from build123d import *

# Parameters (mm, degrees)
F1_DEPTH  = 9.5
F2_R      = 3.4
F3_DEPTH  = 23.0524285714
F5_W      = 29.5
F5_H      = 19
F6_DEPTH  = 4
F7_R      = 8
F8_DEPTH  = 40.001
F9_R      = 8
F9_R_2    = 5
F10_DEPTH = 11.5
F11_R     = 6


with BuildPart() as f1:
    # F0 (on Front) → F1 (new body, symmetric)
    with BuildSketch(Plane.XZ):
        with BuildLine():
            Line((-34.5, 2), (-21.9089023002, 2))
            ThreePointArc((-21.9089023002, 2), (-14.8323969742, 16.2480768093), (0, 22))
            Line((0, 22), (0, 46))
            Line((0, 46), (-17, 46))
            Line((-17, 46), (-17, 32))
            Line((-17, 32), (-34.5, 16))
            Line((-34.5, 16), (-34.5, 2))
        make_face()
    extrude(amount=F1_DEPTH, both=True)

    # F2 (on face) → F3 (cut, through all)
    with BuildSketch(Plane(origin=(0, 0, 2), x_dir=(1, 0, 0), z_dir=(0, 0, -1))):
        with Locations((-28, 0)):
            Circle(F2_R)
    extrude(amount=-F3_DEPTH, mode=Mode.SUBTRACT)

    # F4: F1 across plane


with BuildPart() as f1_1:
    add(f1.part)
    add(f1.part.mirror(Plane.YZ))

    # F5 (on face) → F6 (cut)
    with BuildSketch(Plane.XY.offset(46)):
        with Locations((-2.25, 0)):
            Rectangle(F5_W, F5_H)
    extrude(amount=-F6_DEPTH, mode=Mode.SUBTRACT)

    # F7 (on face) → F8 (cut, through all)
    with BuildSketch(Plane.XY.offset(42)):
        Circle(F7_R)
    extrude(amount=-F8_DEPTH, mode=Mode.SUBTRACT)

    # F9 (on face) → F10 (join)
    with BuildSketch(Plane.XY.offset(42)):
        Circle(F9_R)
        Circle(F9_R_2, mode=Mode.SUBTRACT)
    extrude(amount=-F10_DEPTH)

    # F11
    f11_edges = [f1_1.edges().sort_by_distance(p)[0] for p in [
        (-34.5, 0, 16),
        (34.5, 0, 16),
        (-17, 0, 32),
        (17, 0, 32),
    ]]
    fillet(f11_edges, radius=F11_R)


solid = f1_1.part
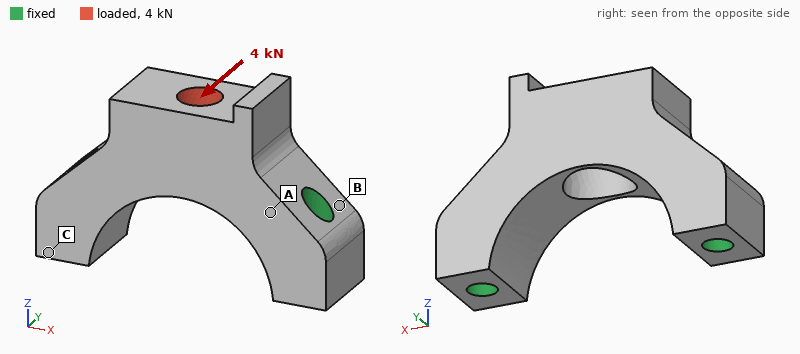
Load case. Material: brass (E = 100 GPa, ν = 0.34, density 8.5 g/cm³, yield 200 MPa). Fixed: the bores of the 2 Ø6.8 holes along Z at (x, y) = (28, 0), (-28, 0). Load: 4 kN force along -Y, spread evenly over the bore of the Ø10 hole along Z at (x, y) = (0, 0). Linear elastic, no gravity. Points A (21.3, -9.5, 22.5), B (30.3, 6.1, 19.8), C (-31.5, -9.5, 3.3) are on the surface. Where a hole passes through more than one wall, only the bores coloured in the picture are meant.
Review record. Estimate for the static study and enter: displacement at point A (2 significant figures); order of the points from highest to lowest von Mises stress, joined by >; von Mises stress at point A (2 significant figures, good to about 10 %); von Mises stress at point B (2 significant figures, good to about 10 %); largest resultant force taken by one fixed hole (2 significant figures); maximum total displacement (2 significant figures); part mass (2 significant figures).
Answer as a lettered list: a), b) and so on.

a) 7.8 µm
b) A > B > C
c) 48 MPa
d) 22 MPa
e) 2.0 kN
f) 37 µm
g) 200 g
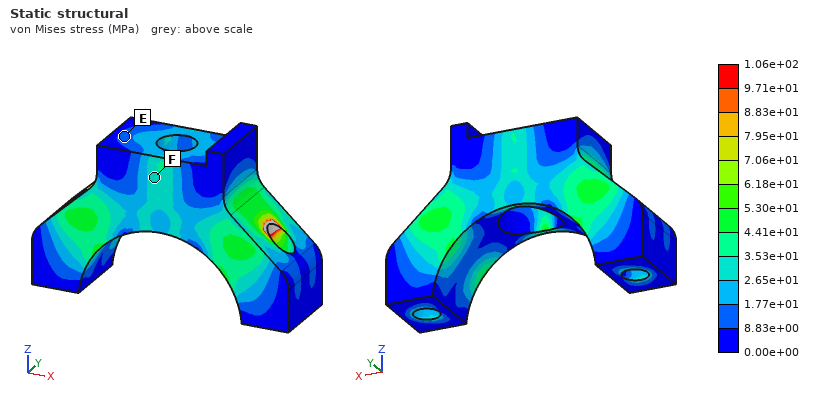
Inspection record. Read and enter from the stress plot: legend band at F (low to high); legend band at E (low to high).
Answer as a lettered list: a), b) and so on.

a) 2.65e+01 to 3.53e+01 MPa
b) 8.83e+00 to 1.77e+01 MPa
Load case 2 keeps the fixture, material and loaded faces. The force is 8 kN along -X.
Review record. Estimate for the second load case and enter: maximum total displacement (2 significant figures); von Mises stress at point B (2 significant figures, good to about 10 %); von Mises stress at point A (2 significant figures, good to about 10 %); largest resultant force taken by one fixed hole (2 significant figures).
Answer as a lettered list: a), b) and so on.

a) 12 µm
b) 13 MPa
c) 15 MPa
d) 4.8 kN
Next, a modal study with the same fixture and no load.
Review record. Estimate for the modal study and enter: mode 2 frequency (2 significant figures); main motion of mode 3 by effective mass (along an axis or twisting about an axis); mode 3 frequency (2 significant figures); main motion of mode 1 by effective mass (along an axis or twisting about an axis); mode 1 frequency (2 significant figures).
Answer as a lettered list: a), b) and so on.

a) 15 kHz
b) along Z
c) 16 kHz
d) along Y
e) 7100 Hz
